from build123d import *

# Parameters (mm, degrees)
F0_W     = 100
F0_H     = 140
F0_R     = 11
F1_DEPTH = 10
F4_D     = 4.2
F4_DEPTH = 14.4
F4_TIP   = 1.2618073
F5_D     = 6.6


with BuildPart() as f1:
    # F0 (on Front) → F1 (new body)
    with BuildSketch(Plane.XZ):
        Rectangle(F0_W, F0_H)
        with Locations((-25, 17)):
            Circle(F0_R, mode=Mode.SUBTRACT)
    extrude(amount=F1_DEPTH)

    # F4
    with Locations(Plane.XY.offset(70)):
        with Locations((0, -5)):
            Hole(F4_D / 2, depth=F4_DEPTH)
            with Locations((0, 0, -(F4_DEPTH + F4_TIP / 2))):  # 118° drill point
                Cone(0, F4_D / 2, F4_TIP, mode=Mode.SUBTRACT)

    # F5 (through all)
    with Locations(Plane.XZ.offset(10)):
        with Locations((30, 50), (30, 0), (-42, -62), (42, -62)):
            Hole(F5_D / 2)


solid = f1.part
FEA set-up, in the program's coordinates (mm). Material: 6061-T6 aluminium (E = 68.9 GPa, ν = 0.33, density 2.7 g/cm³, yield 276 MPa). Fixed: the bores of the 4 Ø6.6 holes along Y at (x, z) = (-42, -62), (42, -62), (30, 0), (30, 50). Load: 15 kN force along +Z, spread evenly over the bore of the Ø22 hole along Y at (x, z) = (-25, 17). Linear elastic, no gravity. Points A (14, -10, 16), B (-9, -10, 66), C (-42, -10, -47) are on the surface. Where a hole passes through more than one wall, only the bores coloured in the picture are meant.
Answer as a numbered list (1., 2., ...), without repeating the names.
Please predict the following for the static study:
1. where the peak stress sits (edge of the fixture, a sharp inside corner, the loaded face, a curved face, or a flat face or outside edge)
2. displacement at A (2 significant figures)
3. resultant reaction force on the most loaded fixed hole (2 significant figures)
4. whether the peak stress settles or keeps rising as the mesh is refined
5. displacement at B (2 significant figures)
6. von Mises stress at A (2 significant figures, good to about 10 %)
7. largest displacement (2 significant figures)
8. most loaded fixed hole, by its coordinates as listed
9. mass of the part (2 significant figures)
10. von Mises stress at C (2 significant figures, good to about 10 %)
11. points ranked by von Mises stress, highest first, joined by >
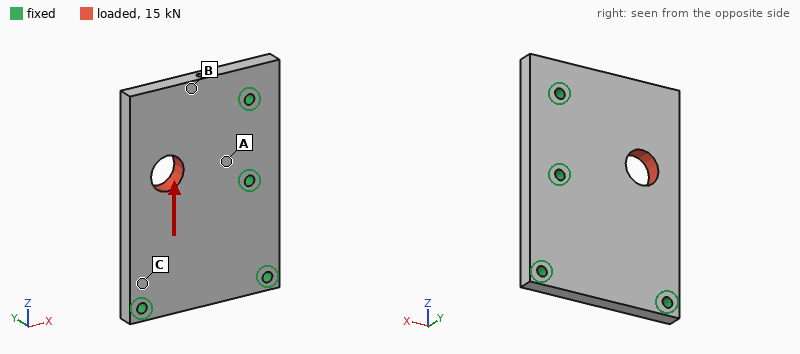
1. edge of the fixture
2. 6.5 µm
3. 6.2 kN
4. keeps rising
5. 23 µm
6. 17 MPa
7. 38 µm
8. (-42, -62)
9. 360 g
10. 30 MPa
11. C > A > B
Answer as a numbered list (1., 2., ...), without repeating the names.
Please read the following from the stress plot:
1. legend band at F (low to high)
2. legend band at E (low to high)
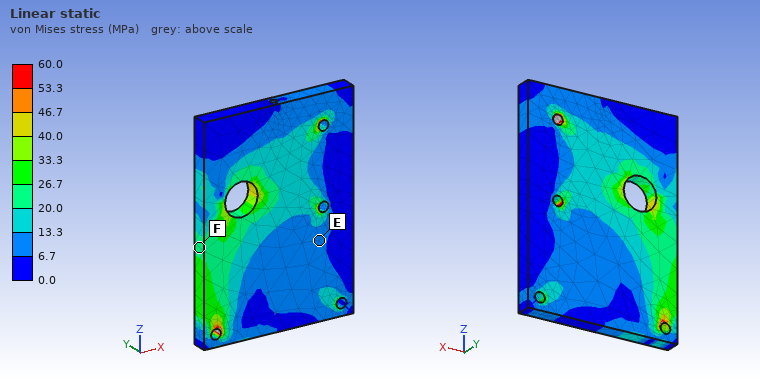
1. 20.0 to 26.7 MPa
2. 6.7 to 13.3 MPa
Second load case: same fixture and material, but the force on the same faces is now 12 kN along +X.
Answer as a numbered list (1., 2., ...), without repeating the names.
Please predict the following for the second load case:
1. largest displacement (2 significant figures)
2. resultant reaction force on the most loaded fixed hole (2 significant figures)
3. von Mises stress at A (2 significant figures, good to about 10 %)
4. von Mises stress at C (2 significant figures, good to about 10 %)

1. 25 µm
2. 5.2 kN
3. 12 MPa
4. 3.9 MPa
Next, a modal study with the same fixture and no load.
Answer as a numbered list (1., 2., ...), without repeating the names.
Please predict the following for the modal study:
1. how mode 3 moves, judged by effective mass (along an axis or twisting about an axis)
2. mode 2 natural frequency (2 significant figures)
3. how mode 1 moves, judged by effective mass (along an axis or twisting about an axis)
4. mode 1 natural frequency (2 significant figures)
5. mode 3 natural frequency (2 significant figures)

1. along Y
2. 3800 Hz
3. along Y
4. 1600 Hz
5. 6200 Hz
